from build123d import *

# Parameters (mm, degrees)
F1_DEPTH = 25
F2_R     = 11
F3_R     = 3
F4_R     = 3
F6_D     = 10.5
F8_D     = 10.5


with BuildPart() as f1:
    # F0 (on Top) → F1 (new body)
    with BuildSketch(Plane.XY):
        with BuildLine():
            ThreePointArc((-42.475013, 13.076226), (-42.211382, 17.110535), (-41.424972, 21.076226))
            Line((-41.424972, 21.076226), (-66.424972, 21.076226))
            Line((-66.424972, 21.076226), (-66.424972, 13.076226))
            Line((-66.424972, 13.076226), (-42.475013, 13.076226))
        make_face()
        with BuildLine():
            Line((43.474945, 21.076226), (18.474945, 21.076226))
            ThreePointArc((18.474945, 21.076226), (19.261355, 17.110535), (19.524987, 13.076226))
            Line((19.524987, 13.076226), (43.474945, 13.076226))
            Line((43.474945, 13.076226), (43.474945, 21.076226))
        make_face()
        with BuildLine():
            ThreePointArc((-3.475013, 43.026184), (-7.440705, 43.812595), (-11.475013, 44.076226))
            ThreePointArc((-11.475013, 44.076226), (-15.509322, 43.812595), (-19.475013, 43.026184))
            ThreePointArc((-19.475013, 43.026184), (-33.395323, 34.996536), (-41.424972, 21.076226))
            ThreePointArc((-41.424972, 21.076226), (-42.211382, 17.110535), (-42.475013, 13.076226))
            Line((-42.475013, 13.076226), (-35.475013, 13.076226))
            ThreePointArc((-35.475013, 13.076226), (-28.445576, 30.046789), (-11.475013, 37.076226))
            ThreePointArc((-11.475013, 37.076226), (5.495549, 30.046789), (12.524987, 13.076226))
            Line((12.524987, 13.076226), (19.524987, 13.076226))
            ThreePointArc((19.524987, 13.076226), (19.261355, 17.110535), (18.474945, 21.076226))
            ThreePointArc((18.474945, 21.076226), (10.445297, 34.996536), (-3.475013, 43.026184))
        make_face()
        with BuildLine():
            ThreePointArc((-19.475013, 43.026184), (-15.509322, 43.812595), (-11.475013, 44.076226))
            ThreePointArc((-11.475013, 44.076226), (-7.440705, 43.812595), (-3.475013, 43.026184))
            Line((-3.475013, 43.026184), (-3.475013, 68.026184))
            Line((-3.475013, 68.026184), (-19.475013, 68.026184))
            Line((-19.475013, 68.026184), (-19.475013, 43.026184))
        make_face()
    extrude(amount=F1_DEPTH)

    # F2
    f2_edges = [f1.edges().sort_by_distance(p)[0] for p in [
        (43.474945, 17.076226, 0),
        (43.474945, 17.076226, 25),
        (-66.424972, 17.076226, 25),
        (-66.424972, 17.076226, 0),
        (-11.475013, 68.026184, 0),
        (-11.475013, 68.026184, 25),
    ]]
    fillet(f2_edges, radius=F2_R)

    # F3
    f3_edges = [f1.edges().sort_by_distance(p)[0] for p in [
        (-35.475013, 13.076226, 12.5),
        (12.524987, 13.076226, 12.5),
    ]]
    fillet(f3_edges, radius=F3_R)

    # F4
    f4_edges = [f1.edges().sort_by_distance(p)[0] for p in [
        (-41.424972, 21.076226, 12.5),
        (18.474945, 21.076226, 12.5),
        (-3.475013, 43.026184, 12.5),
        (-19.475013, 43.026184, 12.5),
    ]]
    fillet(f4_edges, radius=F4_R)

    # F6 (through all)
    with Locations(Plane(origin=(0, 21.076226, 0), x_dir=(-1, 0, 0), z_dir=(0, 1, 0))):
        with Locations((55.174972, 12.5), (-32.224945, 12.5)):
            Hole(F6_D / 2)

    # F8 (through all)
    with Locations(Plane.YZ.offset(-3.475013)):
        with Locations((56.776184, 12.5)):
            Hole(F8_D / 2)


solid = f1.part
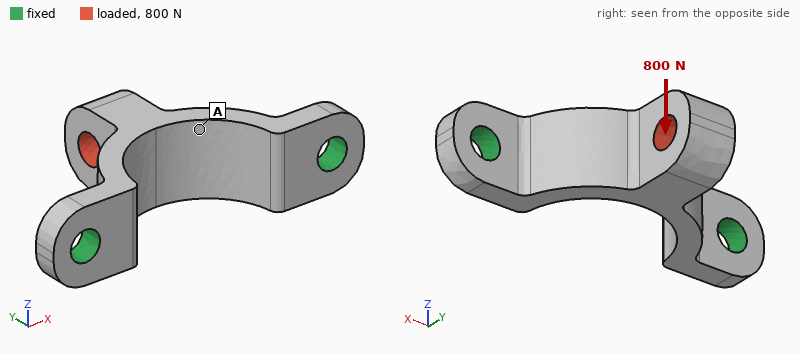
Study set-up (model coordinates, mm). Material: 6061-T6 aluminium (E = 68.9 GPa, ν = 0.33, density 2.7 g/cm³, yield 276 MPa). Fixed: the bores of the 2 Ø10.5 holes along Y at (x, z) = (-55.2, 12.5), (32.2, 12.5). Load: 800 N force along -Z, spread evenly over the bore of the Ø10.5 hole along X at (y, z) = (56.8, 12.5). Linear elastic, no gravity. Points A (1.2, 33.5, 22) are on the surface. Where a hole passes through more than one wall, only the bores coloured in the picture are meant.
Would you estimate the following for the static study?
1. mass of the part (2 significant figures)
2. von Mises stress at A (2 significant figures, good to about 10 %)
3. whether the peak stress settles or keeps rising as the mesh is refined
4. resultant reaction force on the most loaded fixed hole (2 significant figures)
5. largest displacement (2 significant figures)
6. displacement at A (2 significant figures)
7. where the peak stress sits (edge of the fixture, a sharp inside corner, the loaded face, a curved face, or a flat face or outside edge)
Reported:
81 g
15 MPa
keeps rising
400 N
0.13 mm
0.044 mm
edge of the fixture
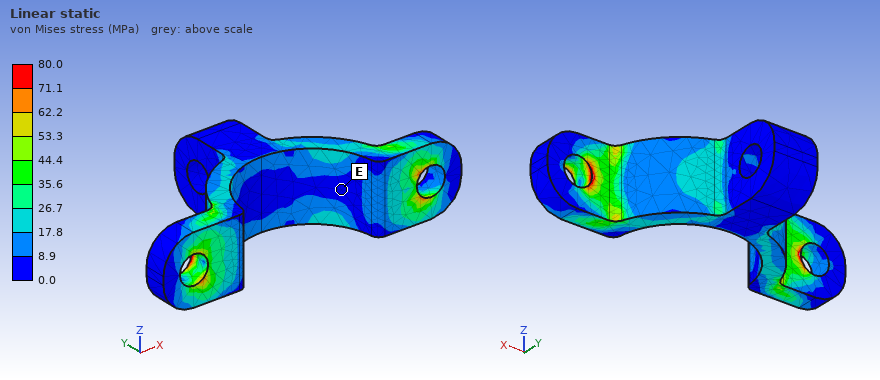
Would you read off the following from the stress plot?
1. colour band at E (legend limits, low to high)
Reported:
0.0 to 8.9 MPa
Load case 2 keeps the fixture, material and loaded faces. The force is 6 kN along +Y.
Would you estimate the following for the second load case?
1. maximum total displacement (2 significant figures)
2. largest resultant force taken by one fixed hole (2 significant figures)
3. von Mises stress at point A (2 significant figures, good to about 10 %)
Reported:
49 µm
4.3 kN
37 MPa
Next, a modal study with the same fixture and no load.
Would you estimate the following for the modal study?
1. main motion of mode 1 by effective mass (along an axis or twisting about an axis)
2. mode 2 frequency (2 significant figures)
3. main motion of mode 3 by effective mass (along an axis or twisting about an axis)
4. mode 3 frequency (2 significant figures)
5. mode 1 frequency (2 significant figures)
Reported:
along Z
7400 Hz
along Y
9100 Hz
2700 Hz
